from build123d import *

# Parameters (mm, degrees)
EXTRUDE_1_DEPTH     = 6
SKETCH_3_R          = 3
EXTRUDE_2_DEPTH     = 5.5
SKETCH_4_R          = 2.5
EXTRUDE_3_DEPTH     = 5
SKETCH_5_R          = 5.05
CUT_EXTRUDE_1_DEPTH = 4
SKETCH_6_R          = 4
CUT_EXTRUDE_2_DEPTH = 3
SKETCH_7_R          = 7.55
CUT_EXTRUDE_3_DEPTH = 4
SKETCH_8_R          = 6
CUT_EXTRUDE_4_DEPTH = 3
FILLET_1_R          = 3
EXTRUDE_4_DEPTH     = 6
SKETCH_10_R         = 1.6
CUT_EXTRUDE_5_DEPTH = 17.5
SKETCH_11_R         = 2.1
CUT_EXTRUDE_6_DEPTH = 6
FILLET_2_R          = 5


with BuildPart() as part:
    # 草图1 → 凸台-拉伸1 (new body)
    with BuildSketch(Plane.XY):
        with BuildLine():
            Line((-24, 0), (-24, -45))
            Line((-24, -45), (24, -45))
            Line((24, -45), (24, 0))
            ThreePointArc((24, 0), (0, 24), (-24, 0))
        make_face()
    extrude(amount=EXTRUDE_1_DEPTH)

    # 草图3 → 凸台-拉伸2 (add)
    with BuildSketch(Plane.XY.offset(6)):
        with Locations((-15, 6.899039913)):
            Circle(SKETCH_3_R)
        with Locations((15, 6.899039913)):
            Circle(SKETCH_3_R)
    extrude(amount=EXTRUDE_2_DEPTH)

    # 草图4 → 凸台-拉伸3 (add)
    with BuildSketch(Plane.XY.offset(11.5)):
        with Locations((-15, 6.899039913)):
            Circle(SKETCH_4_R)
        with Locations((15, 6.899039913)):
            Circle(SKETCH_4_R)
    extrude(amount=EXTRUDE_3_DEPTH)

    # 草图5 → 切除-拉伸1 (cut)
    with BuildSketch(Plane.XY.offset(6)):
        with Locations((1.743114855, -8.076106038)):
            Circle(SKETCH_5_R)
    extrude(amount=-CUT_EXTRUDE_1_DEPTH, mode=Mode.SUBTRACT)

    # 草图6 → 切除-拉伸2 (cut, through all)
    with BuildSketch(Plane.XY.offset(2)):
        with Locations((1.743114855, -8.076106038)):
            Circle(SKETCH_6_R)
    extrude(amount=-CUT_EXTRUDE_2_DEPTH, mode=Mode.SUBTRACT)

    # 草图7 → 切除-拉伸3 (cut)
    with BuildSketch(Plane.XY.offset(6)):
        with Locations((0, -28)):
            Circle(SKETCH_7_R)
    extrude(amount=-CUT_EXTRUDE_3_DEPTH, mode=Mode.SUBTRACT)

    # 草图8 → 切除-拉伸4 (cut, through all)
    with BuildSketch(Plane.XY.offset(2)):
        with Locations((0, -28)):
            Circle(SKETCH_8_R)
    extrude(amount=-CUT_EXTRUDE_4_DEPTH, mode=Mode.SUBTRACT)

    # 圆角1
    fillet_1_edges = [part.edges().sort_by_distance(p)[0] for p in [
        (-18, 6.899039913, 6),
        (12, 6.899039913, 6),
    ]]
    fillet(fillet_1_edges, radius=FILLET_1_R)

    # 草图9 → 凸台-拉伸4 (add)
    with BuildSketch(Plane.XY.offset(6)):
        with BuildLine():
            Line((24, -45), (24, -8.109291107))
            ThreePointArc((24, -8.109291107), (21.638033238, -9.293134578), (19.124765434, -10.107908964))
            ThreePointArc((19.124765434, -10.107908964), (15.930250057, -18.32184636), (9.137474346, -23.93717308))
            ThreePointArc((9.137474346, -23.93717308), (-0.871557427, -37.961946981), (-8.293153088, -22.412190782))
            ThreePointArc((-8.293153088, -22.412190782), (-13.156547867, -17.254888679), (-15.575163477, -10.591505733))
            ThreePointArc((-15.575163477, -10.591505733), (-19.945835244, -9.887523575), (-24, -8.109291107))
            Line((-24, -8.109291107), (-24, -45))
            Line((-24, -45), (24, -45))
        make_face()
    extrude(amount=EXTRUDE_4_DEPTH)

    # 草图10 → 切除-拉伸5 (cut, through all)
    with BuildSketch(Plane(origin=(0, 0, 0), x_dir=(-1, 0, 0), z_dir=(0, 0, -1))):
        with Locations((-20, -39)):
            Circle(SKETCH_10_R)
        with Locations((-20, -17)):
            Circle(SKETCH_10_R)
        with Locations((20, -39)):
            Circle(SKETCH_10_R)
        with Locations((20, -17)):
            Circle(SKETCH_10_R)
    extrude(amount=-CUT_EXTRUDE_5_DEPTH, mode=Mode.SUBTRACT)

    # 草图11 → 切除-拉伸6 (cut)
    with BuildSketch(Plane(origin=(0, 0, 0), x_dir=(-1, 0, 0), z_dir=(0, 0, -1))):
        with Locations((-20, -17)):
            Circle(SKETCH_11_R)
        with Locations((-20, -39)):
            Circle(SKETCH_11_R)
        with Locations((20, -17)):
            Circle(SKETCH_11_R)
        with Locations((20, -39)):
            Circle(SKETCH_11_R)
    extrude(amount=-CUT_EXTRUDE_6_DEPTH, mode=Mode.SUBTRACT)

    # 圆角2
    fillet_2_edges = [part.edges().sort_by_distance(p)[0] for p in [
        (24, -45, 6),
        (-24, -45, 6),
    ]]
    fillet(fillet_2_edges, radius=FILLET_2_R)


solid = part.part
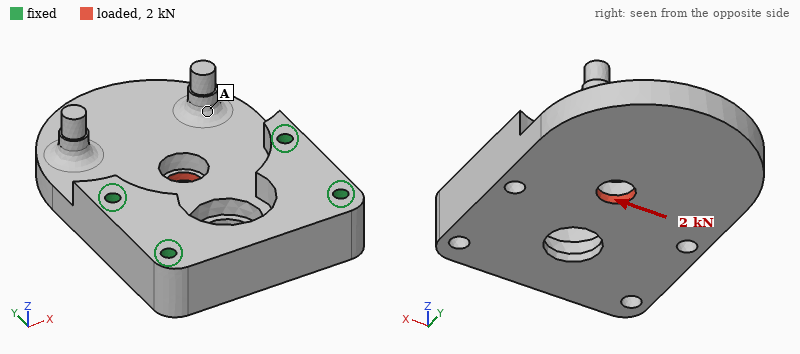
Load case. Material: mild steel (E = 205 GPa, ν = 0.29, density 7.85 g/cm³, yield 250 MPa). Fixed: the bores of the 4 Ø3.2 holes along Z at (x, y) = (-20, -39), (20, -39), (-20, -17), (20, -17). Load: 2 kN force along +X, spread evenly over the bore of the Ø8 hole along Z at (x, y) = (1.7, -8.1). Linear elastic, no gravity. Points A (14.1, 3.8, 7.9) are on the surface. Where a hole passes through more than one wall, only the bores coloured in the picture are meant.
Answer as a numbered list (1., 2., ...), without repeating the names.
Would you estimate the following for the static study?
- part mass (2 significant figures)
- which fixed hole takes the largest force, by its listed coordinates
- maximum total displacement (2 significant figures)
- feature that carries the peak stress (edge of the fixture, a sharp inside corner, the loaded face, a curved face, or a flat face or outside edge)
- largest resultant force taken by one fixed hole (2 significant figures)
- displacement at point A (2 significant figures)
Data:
1. 180 g
2. (-20, -17)
3. 3.3 µm
4. edge of the fixture
5. 980 N
6. 2.5 µm
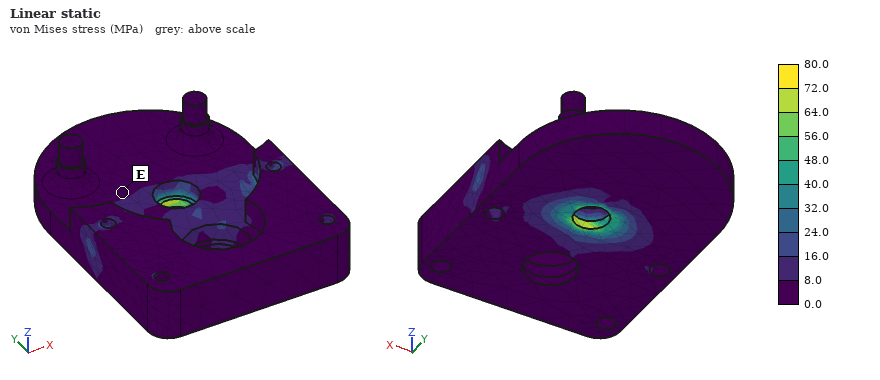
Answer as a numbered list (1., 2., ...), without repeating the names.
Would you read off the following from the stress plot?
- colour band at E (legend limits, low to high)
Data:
1. 0.0 to 8.0 MPa
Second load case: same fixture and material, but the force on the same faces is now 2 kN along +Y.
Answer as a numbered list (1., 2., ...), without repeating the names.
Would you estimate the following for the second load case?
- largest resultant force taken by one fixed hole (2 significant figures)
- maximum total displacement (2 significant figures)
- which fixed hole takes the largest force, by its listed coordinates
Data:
1. 680 N
2. 13 µm
3. (20, -39)
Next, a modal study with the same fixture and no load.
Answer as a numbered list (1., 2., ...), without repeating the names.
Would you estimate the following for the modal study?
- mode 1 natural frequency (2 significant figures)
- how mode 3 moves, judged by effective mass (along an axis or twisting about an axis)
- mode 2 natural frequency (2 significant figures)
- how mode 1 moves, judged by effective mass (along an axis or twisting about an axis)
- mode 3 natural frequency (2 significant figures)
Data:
1. 3200 Hz
2. along X
3. 8400 Hz
4. along Z
5. 12 kHz
